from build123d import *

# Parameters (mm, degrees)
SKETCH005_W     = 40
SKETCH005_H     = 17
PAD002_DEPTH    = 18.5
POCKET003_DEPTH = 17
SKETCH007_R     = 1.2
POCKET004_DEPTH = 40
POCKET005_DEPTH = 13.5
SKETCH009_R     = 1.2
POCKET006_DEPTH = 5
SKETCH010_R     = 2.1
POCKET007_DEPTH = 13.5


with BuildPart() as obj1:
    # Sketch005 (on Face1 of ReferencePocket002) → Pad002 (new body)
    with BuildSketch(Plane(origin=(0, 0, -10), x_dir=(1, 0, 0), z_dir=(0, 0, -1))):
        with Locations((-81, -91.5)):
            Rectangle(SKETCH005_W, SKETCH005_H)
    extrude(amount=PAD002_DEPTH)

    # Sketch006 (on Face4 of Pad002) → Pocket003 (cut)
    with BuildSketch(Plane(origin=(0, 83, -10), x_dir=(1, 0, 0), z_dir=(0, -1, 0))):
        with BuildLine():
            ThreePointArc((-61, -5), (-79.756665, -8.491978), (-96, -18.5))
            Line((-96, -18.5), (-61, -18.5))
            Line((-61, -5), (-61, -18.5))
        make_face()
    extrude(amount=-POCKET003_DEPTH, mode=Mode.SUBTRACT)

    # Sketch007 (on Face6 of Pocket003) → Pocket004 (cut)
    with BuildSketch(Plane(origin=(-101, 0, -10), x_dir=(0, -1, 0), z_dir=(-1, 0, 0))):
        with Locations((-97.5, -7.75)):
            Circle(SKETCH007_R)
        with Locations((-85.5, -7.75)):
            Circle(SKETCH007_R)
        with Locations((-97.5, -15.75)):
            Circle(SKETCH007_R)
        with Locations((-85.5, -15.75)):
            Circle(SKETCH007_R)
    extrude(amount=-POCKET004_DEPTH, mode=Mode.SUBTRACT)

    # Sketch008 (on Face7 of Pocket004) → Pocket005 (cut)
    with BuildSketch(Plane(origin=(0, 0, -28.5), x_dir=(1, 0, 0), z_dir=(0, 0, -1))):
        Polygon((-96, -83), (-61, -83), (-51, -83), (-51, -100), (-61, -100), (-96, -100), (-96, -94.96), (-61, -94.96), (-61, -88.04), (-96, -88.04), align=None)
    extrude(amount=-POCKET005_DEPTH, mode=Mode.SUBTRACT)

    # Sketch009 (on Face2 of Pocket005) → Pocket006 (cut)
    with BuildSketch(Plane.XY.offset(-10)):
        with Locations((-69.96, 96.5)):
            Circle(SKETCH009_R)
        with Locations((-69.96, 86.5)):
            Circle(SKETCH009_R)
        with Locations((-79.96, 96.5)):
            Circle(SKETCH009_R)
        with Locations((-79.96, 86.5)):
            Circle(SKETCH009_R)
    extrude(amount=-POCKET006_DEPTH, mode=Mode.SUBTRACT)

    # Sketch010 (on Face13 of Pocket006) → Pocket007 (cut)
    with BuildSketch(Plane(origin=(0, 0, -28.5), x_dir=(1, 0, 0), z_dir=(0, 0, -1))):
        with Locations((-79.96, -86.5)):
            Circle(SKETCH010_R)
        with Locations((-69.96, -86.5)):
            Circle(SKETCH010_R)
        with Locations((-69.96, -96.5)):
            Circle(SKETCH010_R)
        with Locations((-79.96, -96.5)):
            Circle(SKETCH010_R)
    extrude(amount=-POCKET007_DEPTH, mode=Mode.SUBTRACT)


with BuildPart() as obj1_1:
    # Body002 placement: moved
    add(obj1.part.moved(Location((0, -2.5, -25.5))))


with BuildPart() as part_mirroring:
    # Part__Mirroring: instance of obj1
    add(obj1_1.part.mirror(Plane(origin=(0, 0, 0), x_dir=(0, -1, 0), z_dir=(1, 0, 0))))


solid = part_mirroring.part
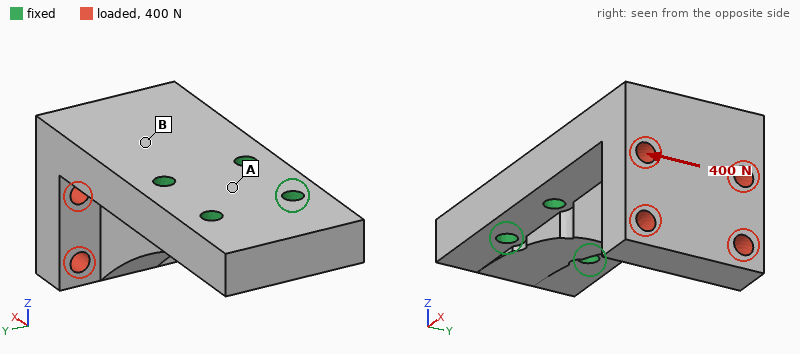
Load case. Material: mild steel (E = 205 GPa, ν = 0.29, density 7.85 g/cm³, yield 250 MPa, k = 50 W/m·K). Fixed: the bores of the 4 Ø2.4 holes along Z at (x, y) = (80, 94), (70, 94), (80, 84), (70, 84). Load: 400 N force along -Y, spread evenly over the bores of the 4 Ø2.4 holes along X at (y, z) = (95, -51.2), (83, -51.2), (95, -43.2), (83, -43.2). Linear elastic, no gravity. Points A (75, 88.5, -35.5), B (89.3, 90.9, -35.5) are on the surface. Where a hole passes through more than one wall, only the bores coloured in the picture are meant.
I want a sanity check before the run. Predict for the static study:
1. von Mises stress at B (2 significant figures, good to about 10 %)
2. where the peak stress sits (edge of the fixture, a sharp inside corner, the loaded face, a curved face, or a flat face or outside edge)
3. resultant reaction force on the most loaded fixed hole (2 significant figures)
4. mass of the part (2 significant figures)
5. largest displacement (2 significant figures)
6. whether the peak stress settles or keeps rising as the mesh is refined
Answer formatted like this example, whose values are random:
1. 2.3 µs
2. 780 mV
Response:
1. 11 MPa
2. edge of the fixture
3. 700 N
4. 42 g
5. 11 µm
6. keeps rising
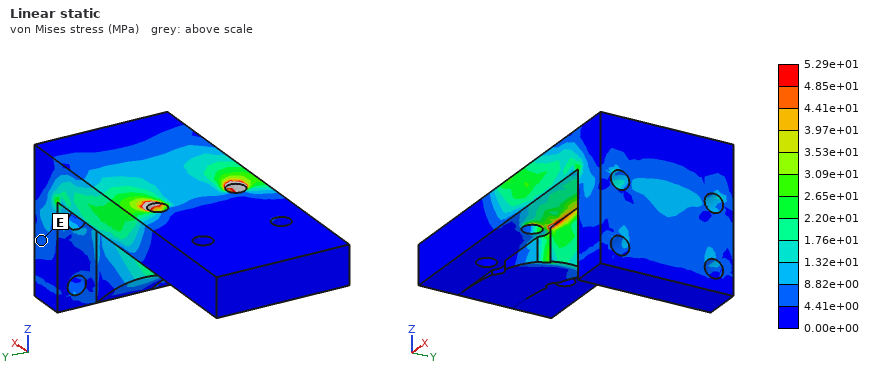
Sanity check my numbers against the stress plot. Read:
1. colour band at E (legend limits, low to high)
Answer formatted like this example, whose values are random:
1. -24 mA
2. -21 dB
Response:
1. 4.41e+00 to 8.82e+00 MPa
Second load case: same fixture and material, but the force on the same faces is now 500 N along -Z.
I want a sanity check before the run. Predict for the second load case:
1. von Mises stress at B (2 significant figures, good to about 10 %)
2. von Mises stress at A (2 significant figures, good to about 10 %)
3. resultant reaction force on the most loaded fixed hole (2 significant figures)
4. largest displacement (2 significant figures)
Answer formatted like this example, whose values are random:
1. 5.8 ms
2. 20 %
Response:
1. 20 MPa
2. 14 MPa
3. 490 N
4. 18 µm
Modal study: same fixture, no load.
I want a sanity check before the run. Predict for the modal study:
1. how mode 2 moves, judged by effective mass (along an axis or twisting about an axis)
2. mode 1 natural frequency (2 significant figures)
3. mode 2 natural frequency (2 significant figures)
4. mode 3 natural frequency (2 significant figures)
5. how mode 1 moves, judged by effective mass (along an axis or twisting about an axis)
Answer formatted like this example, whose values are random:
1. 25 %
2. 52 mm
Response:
1. along Y
2. 7200 Hz
3. 11 kHz
4. 19 kHz
5. along Z
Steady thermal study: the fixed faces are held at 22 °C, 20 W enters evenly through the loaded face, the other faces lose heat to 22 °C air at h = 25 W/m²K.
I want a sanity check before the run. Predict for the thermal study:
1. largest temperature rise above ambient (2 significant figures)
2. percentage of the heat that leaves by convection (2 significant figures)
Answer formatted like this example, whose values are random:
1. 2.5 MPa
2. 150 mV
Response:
1. 76 K
2. 9.6 %
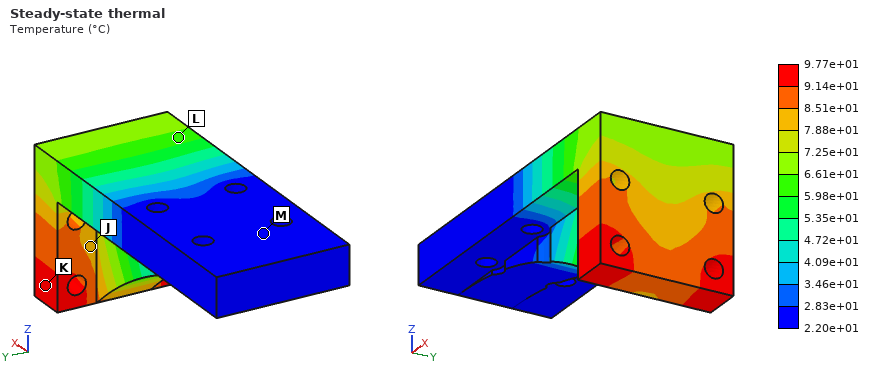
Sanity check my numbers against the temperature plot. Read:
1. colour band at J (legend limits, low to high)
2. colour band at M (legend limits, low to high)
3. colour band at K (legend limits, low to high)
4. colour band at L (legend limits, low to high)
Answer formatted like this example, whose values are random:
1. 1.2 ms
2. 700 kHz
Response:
1. 7.88e+01 to 8.51e+01 °C
2. 2.20e+01 to 2.83e+01 °C
3. 9.14e+01 to 9.77e+01 °C
4. 5.98e+01 to 6.61e+01 °C
